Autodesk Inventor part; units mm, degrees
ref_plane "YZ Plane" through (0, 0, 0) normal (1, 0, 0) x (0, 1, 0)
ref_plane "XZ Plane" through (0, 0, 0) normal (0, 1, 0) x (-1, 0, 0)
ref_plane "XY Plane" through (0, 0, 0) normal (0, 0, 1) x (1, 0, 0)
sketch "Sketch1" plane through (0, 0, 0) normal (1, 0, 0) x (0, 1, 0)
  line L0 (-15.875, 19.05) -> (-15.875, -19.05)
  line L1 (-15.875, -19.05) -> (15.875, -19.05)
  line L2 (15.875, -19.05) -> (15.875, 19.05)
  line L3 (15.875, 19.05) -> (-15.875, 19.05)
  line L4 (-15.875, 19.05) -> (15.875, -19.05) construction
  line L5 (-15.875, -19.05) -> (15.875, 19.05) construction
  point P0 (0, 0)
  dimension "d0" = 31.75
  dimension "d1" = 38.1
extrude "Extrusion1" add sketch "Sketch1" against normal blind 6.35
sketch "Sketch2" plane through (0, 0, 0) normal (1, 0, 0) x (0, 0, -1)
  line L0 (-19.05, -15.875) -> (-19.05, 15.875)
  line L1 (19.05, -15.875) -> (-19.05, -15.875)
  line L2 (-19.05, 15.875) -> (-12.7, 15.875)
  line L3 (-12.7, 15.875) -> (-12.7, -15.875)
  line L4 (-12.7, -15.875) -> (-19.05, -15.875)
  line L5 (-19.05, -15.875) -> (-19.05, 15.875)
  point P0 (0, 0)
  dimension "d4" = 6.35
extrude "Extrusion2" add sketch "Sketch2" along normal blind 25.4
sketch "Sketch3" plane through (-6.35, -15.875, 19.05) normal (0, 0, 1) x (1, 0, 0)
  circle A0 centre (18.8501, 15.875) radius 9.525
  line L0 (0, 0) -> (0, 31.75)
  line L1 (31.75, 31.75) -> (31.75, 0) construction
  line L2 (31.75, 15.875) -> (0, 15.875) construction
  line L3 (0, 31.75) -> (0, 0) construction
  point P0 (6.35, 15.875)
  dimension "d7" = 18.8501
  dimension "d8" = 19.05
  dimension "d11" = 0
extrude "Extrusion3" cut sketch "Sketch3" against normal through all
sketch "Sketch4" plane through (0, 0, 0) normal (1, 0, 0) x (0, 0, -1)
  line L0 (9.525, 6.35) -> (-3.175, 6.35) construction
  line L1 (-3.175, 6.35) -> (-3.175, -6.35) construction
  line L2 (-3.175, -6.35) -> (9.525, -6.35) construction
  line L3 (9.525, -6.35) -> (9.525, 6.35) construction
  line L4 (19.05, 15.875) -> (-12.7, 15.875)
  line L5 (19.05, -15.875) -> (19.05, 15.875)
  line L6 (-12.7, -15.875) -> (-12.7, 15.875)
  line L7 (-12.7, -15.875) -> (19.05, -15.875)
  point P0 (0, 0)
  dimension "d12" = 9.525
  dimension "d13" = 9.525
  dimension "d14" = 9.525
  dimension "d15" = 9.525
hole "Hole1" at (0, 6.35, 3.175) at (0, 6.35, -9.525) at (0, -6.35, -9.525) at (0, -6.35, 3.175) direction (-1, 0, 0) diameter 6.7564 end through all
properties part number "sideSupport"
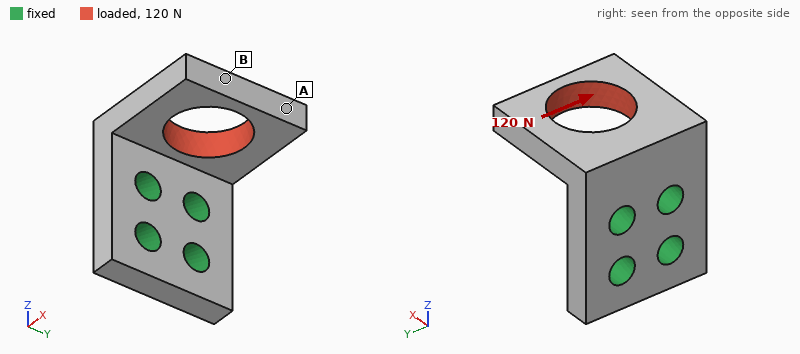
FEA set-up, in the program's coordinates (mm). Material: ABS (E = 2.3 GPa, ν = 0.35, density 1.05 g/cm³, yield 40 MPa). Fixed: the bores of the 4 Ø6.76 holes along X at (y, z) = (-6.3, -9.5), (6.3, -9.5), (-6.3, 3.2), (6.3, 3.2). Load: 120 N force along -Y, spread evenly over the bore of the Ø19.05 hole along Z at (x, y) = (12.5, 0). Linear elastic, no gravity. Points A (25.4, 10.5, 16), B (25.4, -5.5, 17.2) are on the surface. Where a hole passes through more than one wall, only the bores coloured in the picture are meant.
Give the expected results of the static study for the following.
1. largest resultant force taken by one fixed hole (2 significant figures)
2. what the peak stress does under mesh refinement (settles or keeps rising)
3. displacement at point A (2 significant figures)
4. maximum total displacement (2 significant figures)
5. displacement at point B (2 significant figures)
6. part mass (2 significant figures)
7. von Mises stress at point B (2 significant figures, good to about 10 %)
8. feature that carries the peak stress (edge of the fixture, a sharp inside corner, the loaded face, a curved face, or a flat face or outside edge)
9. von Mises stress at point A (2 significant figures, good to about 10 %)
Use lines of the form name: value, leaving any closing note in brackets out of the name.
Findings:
largest resultant force taken by one fixed hole: 120 N
what the peak stress does under mesh refinement: keeps rising
displacement at point A: 0.21 mm
maximum total displacement: 0.23 mm
displacement at point B: 0.20 mm
part mass: 11 g
von Mises stress at point B: 3.3 MPa
feature that carries the peak stress: edge of the fixture
von Mises stress at point A: 1.5 MPa
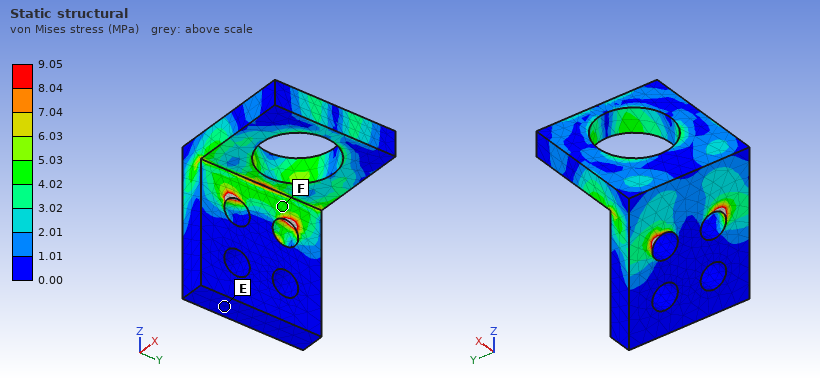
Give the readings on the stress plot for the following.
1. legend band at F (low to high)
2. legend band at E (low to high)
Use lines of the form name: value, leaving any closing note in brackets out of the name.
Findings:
legend band at F: 4.02 to 5.03 MPa
legend band at E: 0.00 to 1.01 MPa
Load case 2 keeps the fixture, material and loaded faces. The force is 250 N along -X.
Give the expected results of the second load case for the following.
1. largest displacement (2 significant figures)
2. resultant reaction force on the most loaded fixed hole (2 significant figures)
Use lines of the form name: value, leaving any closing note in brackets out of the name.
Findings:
largest displacement: 0.32 mm
resultant reaction force on the most loaded fixed hole: 140 N
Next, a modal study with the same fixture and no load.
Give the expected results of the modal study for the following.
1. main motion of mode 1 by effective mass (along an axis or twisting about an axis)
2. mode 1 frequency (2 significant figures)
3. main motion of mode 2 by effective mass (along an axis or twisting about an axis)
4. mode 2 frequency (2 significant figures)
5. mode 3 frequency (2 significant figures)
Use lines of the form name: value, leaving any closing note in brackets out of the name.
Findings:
main motion of mode 1 by effective mass: along Z
mode 1 frequency: 1300 Hz
main motion of mode 2 by effective mass: along Y
mode 2 frequency: 2100 Hz
mode 3 frequency: 2800 Hz
